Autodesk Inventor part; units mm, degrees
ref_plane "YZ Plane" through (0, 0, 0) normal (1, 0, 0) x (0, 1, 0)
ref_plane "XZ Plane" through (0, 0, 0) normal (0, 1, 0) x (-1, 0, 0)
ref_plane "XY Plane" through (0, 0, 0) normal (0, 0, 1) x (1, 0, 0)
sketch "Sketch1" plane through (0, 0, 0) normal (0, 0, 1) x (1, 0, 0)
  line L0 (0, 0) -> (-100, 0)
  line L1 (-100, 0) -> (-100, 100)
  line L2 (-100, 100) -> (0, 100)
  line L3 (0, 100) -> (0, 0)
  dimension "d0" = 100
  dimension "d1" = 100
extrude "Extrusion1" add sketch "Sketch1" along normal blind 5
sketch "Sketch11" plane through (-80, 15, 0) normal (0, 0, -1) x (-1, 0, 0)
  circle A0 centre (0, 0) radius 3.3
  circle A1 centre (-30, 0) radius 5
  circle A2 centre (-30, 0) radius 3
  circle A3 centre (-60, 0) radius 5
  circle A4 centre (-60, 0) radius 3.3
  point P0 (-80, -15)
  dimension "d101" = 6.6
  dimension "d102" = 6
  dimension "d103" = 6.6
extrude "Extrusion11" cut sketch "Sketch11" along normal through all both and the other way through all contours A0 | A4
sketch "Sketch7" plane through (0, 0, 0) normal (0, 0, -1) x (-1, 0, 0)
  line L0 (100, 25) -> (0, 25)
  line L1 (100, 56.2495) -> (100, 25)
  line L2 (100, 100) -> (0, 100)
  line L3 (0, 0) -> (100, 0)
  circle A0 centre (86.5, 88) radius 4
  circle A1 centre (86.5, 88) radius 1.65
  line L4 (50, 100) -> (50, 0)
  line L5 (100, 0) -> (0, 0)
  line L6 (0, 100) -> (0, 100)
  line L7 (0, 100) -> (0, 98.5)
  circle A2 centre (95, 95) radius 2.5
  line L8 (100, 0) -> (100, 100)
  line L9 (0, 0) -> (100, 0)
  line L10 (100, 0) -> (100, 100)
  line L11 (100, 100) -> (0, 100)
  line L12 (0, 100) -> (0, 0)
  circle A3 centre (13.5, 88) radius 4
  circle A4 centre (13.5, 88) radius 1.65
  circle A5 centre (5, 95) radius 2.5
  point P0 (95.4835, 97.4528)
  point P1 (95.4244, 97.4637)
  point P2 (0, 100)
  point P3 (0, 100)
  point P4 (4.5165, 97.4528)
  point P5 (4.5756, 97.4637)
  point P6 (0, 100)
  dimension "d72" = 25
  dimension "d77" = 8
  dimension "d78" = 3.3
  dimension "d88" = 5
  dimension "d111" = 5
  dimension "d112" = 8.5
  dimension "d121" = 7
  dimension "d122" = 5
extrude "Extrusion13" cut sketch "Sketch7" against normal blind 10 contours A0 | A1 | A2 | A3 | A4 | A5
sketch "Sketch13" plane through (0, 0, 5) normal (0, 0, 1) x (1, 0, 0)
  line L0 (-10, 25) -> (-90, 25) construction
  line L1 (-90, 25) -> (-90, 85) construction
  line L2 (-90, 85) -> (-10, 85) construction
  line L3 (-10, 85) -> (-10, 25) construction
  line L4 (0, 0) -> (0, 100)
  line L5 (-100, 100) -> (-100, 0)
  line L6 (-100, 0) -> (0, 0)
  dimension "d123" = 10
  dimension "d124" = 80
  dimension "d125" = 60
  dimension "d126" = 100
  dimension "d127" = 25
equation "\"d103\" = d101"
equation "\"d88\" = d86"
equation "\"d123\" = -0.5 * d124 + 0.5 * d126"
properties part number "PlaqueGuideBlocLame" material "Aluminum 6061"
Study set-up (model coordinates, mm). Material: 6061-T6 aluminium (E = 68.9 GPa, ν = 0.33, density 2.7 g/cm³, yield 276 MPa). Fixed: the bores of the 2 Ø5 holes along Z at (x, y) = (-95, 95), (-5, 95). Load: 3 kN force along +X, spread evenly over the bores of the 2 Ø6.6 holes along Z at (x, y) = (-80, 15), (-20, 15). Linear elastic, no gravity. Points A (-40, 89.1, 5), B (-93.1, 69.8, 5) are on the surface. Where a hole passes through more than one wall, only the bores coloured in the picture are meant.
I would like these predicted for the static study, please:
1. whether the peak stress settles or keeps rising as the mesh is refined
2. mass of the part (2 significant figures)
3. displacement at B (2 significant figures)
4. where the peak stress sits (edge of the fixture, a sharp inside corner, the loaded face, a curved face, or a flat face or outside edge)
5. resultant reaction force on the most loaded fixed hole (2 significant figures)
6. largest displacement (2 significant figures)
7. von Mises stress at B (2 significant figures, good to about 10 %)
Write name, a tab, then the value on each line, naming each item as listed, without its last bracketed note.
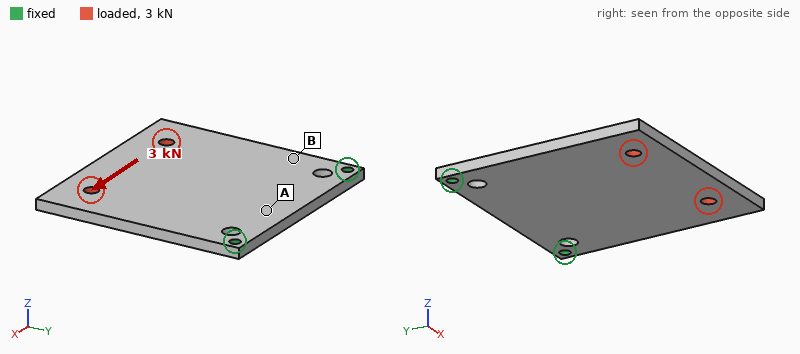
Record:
whether the peak stress settles or keeps rising as the mesh is refined	keeps rising
mass of the part	130 g
displacement at B	20 µm
where the peak stress sits	edge of the fixture
resultant reaction force on the most loaded fixed hole	3.0 kN
largest displacement	63 µm
von Mises stress at B	23 MPa
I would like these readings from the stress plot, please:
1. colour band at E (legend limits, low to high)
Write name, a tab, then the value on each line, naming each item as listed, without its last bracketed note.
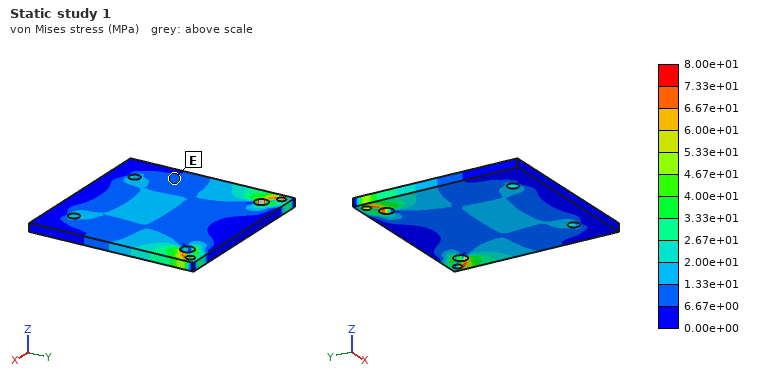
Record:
colour band at E	6.67e+00 to 1.33e+01 MPa
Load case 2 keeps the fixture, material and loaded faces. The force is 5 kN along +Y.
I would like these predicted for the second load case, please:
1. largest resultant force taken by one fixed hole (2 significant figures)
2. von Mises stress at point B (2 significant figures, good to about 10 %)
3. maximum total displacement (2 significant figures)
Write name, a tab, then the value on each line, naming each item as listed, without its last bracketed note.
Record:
largest resultant force taken by one fixed hole	2.6 kN
von Mises stress at point B	22 MPa
maximum total displacement	28 µm
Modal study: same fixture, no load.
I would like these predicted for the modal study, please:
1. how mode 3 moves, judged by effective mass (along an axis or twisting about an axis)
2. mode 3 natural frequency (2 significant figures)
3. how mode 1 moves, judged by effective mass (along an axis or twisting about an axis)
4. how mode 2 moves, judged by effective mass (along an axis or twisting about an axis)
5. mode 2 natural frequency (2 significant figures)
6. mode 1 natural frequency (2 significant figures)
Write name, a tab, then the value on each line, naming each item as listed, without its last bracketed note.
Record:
how mode 3 moves, judged by effective mass	along Z
mode 3 natural frequency	2200 Hz
how mode 1 moves, judged by effective mass	along Z
how mode 2 moves, judged by effective mass	twisting about Y
mode 2 natural frequency	1000 Hz
mode 1 natural frequency	320 Hz
